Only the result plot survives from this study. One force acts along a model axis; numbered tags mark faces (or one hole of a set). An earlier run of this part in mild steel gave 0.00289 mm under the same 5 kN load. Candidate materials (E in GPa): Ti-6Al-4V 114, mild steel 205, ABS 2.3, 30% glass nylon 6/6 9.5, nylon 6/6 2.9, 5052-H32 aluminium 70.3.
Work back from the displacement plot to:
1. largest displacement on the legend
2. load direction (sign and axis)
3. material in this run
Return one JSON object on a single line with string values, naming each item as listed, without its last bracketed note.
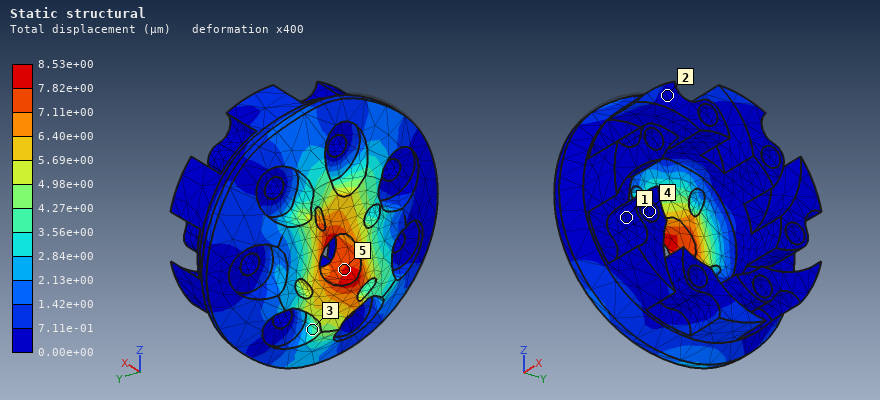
{"largest displacement on the legend": "8.53e+00 µm", "load direction": "-Z", "material in this run": "5052-H32 aluminium"}
